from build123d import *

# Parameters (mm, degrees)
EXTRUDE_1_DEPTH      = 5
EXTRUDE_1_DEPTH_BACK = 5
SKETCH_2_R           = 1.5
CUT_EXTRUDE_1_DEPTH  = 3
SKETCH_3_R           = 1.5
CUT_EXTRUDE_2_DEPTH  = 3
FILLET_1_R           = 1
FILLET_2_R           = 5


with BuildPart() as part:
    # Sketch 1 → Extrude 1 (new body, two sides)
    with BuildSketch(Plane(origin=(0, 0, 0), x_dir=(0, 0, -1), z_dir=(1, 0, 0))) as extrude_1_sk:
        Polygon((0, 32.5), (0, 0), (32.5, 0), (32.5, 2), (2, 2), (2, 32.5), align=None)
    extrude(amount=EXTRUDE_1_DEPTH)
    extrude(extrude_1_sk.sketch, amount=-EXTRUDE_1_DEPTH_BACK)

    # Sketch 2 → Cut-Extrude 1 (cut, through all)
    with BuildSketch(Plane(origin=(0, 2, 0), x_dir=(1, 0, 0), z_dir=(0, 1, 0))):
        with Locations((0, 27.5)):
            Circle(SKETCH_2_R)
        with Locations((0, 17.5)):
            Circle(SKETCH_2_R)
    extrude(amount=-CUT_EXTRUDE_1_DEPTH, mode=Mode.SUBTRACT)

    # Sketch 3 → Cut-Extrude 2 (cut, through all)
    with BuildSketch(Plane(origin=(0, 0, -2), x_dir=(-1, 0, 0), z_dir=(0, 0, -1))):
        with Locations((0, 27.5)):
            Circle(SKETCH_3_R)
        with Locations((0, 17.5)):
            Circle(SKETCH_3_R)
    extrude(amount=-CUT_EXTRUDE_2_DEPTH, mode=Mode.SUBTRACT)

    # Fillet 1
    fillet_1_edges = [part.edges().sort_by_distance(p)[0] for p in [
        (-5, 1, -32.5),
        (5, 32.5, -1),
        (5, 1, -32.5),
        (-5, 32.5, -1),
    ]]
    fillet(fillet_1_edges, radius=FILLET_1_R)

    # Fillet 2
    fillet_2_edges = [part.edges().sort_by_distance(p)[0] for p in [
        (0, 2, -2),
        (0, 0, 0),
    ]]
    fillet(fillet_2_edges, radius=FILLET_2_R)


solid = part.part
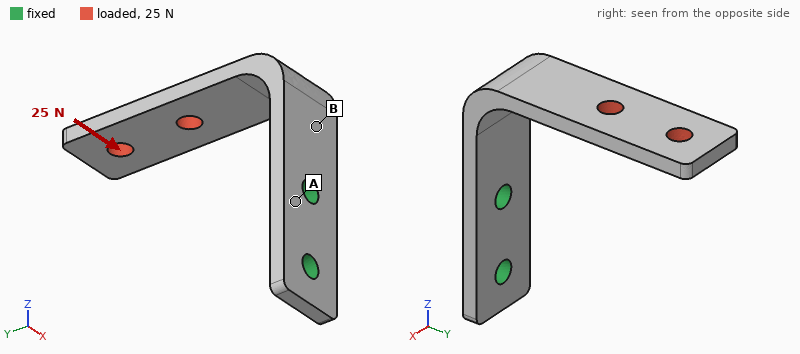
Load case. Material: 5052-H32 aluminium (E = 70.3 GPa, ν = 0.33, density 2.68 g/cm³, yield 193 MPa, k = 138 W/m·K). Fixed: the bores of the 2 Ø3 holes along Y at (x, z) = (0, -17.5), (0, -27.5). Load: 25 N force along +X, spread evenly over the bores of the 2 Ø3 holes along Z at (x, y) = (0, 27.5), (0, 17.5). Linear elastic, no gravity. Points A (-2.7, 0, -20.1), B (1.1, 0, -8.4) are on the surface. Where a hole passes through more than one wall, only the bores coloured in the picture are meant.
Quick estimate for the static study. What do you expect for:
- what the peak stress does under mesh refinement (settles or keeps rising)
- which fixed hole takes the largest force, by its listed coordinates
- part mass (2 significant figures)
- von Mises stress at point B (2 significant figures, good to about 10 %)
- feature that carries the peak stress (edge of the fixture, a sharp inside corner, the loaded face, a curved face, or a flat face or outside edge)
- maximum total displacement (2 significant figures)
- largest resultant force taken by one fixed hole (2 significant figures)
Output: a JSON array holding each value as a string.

["keeps rising", "(0, -17.5)", "3.2 g", "63 MPa", "edge of the fixture", "0.32 mm", "46 N"]
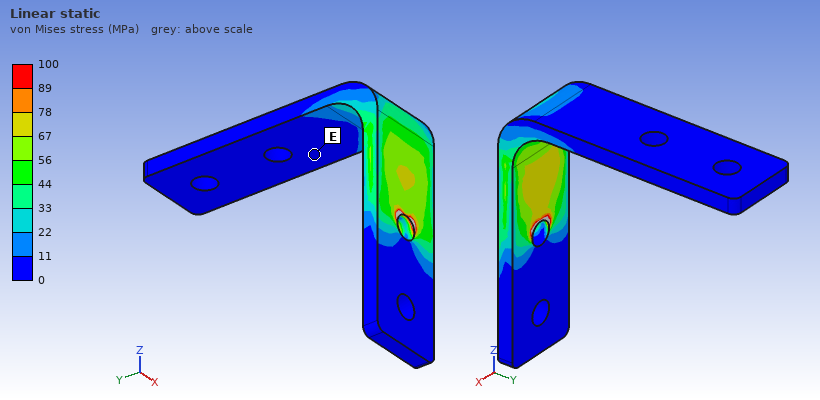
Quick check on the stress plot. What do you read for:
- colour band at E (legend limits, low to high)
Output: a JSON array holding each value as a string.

["0 to 11 MPa"]
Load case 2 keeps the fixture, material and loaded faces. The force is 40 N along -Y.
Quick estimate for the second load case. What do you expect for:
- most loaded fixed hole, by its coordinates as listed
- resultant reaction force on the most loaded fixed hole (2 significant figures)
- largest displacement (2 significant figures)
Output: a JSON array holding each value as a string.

["(0, -17.5)", "47 N", "0.34 mm"]
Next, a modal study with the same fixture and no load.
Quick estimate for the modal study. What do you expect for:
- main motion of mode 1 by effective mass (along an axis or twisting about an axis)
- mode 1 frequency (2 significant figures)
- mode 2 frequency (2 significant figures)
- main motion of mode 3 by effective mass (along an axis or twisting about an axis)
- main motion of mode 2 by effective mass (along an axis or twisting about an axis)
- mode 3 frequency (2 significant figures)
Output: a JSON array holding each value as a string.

["along Z", "1100 Hz", "1600 Hz", "along Y", "along X", "3700 Hz"]
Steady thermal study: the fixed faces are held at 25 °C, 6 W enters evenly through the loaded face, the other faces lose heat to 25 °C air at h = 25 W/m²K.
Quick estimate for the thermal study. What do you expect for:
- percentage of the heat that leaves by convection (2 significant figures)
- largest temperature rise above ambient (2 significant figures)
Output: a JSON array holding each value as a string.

["17 %", "67 K"]
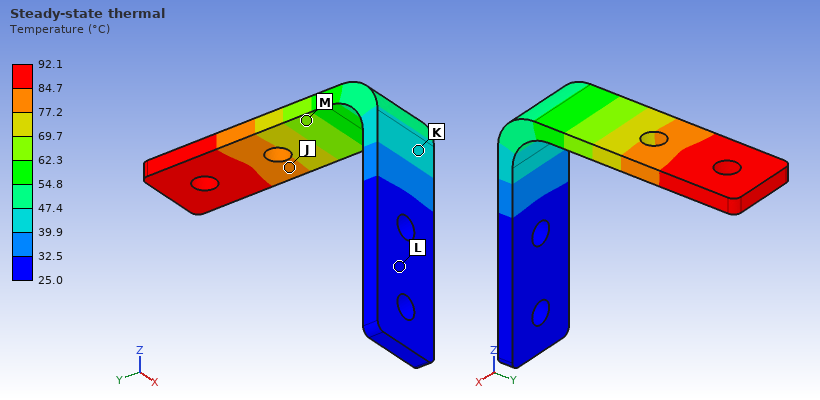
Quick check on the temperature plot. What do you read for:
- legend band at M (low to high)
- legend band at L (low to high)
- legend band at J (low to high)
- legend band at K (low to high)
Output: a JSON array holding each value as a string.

["62.3 to 69.7 °C", "25.0 to 32.5 °C", "77.2 to 84.7 °C", "39.9 to 47.4 °C"]
